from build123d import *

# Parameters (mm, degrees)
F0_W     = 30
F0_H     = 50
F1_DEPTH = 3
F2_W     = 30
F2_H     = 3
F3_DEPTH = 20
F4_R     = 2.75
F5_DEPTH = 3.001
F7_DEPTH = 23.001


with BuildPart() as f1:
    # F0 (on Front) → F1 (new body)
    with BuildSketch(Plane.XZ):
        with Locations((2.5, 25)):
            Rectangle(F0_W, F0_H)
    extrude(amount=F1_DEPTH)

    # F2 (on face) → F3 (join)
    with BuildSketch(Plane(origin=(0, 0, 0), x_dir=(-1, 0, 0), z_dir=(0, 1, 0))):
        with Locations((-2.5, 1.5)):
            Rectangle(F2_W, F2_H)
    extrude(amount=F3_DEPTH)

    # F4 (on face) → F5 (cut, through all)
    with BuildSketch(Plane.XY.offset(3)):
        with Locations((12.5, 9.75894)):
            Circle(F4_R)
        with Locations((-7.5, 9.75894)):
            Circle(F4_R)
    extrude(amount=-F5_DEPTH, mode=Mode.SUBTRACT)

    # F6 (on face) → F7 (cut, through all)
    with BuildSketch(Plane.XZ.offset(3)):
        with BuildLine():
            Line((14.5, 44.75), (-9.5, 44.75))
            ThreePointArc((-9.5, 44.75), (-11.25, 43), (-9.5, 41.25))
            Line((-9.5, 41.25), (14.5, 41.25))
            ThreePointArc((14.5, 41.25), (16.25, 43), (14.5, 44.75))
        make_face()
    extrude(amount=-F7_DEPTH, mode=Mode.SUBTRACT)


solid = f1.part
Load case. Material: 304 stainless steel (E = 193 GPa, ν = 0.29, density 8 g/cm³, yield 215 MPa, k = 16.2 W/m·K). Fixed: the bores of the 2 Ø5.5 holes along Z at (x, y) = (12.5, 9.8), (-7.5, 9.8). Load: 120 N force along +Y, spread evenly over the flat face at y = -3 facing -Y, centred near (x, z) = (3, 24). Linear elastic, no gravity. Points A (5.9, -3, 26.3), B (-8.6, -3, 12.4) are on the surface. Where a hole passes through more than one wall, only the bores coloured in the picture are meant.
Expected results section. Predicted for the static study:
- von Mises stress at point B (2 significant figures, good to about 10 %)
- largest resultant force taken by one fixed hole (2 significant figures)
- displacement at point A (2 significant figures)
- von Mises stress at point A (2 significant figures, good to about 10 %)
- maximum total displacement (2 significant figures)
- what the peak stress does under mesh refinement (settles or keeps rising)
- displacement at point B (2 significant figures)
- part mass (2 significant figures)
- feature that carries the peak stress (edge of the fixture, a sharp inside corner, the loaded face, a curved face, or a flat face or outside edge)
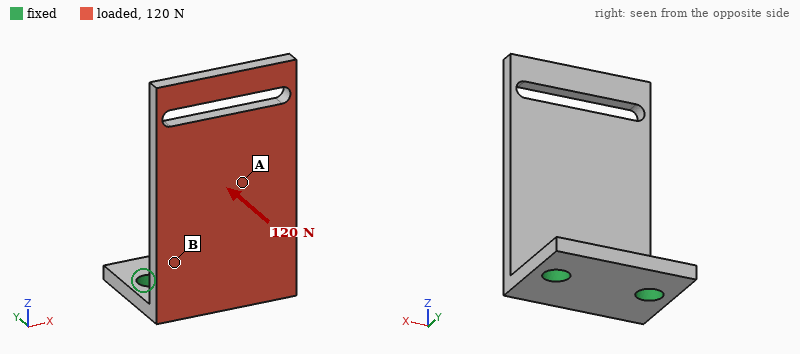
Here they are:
35 MPa
64 N
0.086 mm
12 MPa
0.20 mm
keeps rising
0.032 mm
47 g
edge of the fixture
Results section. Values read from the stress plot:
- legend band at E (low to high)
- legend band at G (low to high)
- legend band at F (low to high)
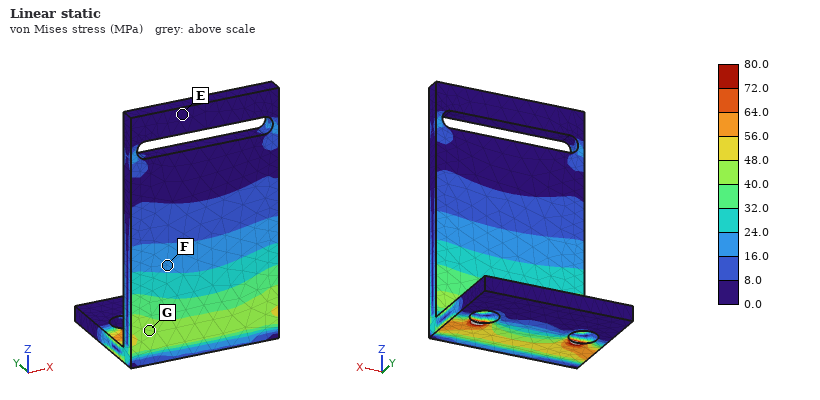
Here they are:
0.0 to 8.0 MPa
40.0 to 48.0 MPa
16.0 to 24.0 MPa
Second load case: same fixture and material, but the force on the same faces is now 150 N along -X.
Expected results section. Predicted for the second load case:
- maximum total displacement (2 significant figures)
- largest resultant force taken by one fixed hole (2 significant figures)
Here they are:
22 µm
190 N
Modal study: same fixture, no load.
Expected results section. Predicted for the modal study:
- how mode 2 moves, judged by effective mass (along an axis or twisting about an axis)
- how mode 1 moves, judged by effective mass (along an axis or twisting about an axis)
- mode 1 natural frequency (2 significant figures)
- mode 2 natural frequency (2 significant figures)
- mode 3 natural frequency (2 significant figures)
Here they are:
along X
along Y
850 Hz
2600 Hz
3700 Hz
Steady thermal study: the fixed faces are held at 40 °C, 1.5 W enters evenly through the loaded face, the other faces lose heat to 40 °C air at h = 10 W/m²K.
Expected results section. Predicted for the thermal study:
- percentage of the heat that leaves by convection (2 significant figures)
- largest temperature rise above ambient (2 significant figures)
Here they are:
26 %
26 K
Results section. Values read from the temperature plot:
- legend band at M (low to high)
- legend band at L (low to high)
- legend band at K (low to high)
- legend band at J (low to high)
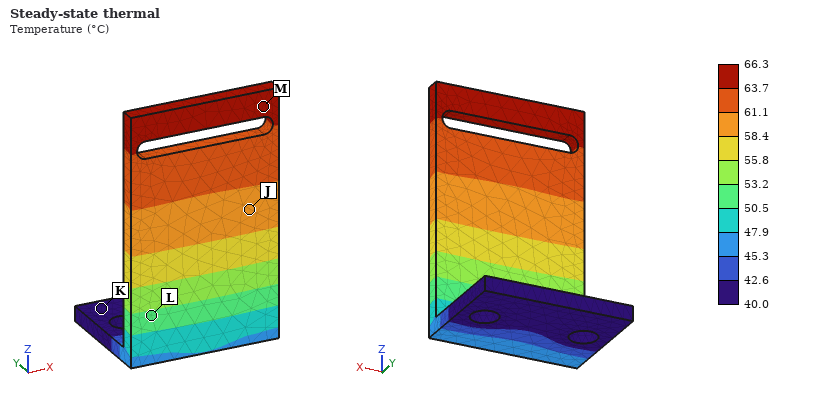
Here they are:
63.7 to 66.3 °C
50.5 to 53.2 °C
40.0 to 42.6 °C
58.4 to 61.1 °C
